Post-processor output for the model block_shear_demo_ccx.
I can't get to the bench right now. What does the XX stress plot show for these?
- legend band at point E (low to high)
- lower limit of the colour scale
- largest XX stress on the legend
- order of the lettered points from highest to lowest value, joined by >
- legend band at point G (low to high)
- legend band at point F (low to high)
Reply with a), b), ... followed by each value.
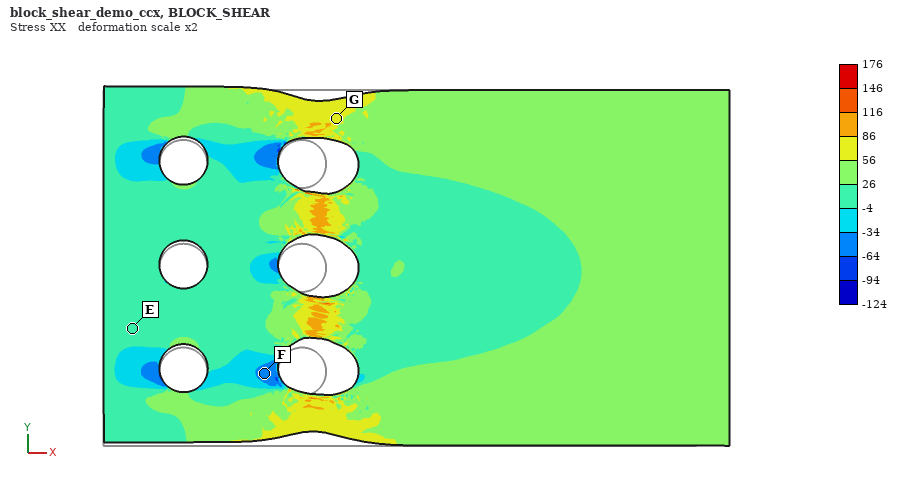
a) -4 to 26
b) -124
c) 176
d) G > E > F
e) 56 to 86
f) -64 to -34
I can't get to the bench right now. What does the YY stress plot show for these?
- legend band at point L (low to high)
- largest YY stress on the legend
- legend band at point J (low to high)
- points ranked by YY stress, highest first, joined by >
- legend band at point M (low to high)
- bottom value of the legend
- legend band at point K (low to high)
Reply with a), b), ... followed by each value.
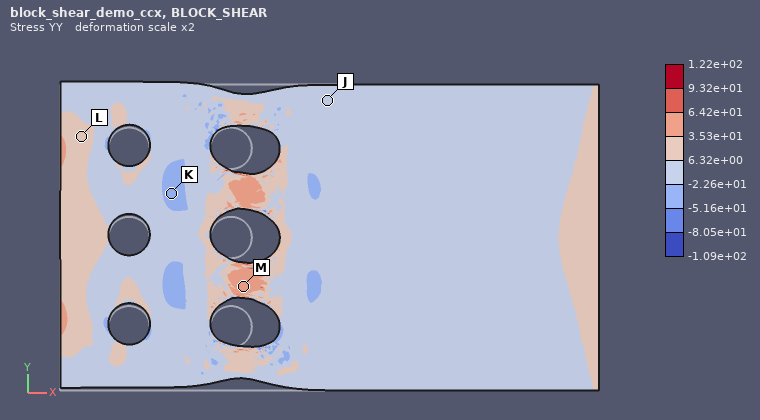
a) 6.32e+00 to 3.53e+01
b) 1.22e+02
c) -2.26e+01 to 6.32e+00
d) M > L > J > K
e) 3.53e+01 to 6.42e+01
f) -1.09e+02
g) -5.16e+01 to -2.26e+01
